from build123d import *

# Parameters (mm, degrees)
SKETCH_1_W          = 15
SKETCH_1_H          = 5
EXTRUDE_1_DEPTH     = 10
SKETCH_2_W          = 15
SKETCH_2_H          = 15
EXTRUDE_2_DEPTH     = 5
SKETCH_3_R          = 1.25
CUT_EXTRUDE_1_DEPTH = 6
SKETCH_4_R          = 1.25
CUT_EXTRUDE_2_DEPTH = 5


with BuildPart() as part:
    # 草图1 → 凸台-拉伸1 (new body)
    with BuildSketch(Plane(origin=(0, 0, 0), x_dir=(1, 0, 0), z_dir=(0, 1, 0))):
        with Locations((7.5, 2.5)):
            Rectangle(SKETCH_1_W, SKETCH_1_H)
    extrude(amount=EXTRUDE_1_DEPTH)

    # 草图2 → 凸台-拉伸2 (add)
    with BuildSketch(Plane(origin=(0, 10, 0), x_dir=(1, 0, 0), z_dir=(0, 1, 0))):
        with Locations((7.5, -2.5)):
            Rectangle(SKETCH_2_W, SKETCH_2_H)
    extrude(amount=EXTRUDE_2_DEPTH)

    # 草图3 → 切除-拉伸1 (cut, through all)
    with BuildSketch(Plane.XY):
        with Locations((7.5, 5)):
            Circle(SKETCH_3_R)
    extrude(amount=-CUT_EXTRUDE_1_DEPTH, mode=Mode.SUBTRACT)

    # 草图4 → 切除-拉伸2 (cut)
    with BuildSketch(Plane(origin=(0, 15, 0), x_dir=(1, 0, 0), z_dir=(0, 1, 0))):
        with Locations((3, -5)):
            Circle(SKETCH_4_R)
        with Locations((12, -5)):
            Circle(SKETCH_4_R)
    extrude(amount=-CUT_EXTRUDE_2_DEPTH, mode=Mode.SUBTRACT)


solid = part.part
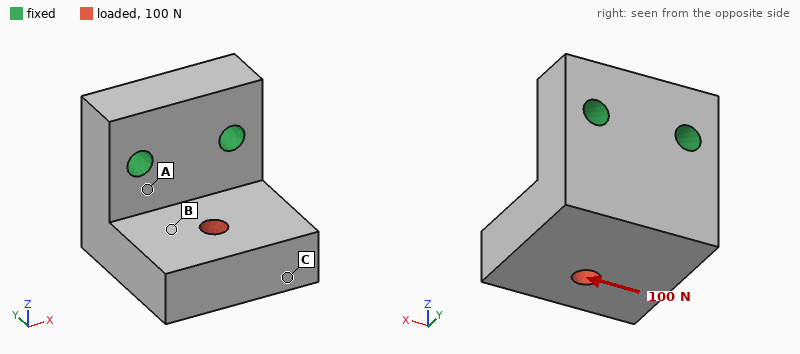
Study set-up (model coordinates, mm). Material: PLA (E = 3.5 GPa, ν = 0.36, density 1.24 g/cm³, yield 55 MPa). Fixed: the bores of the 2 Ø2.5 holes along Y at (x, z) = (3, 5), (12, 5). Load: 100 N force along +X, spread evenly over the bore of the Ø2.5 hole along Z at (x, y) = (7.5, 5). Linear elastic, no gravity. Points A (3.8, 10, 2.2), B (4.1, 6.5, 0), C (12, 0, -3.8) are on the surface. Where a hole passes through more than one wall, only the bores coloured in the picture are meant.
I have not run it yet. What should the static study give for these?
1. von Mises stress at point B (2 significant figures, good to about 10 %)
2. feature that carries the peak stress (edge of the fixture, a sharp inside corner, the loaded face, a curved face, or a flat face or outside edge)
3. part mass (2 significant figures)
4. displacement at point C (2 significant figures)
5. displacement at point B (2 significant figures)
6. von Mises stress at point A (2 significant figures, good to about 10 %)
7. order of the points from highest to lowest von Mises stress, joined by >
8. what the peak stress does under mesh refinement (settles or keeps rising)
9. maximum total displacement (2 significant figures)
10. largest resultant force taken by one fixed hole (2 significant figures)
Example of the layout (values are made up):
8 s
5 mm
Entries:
3.9 MPa
edge of the fixture
2.2 g
65 µm
38 µm
7.8 MPa
A > B > C
keeps rising
72 µm
100 N
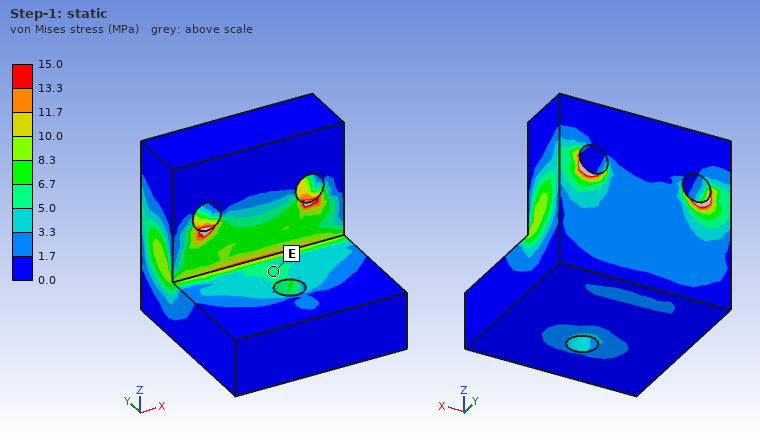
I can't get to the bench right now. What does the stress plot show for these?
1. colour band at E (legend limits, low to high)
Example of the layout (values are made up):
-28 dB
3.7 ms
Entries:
5.0 to 6.7 MPa
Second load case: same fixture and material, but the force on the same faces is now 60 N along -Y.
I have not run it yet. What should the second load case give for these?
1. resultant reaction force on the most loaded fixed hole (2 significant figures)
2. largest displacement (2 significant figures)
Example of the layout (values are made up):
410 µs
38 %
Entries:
30 N
49 µm
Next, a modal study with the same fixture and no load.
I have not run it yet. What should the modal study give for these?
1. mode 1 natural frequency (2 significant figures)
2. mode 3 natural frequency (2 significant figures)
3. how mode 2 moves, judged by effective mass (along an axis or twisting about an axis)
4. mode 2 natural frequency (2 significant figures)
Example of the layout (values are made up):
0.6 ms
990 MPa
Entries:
4500 Hz
12 kHz
along X
6800 Hz
